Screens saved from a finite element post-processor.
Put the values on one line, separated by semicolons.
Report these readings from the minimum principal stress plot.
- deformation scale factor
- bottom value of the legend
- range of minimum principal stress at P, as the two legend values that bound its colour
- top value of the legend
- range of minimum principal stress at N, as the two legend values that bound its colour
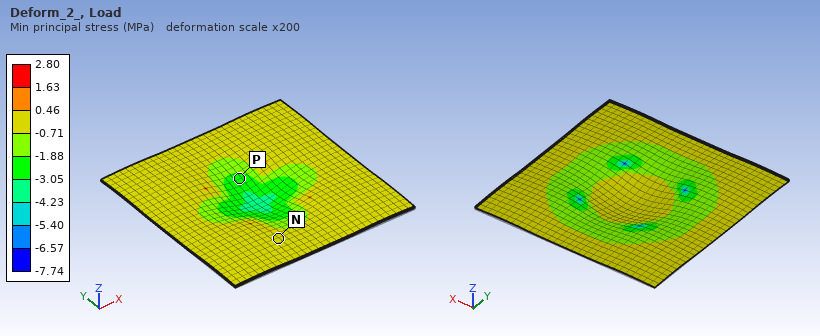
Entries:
200; -7.74 MPa; -3.05 to -1.88 MPa; 2.80 MPa; -0.71 to 0.46 MPa
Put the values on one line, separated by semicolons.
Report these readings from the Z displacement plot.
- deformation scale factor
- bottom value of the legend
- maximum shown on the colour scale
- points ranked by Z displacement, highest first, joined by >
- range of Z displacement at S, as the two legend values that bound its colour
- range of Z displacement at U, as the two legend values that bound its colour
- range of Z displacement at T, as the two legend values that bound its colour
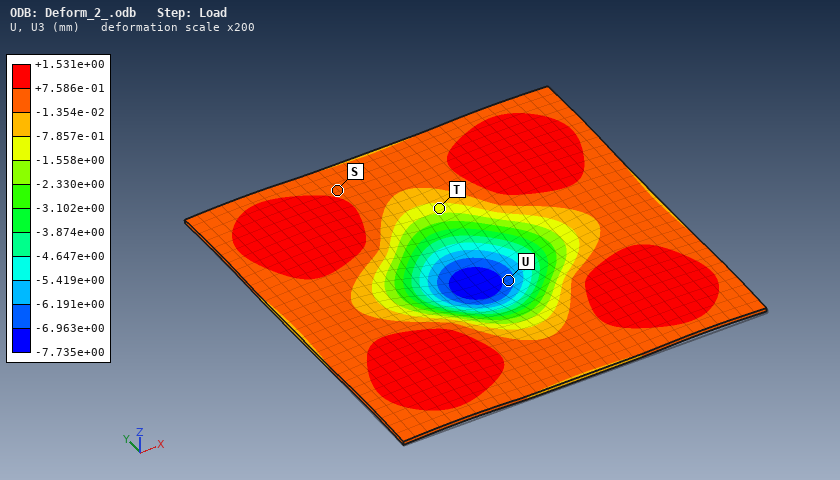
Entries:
200; -7.735e+00 mm; +1.531e+00 mm; S > T > U; -1.354e-02 to +7.586e-01 mm; -6.963e+00 to -6.191e+00 mm; -1.558e+00 to -7.857e-01 mm
